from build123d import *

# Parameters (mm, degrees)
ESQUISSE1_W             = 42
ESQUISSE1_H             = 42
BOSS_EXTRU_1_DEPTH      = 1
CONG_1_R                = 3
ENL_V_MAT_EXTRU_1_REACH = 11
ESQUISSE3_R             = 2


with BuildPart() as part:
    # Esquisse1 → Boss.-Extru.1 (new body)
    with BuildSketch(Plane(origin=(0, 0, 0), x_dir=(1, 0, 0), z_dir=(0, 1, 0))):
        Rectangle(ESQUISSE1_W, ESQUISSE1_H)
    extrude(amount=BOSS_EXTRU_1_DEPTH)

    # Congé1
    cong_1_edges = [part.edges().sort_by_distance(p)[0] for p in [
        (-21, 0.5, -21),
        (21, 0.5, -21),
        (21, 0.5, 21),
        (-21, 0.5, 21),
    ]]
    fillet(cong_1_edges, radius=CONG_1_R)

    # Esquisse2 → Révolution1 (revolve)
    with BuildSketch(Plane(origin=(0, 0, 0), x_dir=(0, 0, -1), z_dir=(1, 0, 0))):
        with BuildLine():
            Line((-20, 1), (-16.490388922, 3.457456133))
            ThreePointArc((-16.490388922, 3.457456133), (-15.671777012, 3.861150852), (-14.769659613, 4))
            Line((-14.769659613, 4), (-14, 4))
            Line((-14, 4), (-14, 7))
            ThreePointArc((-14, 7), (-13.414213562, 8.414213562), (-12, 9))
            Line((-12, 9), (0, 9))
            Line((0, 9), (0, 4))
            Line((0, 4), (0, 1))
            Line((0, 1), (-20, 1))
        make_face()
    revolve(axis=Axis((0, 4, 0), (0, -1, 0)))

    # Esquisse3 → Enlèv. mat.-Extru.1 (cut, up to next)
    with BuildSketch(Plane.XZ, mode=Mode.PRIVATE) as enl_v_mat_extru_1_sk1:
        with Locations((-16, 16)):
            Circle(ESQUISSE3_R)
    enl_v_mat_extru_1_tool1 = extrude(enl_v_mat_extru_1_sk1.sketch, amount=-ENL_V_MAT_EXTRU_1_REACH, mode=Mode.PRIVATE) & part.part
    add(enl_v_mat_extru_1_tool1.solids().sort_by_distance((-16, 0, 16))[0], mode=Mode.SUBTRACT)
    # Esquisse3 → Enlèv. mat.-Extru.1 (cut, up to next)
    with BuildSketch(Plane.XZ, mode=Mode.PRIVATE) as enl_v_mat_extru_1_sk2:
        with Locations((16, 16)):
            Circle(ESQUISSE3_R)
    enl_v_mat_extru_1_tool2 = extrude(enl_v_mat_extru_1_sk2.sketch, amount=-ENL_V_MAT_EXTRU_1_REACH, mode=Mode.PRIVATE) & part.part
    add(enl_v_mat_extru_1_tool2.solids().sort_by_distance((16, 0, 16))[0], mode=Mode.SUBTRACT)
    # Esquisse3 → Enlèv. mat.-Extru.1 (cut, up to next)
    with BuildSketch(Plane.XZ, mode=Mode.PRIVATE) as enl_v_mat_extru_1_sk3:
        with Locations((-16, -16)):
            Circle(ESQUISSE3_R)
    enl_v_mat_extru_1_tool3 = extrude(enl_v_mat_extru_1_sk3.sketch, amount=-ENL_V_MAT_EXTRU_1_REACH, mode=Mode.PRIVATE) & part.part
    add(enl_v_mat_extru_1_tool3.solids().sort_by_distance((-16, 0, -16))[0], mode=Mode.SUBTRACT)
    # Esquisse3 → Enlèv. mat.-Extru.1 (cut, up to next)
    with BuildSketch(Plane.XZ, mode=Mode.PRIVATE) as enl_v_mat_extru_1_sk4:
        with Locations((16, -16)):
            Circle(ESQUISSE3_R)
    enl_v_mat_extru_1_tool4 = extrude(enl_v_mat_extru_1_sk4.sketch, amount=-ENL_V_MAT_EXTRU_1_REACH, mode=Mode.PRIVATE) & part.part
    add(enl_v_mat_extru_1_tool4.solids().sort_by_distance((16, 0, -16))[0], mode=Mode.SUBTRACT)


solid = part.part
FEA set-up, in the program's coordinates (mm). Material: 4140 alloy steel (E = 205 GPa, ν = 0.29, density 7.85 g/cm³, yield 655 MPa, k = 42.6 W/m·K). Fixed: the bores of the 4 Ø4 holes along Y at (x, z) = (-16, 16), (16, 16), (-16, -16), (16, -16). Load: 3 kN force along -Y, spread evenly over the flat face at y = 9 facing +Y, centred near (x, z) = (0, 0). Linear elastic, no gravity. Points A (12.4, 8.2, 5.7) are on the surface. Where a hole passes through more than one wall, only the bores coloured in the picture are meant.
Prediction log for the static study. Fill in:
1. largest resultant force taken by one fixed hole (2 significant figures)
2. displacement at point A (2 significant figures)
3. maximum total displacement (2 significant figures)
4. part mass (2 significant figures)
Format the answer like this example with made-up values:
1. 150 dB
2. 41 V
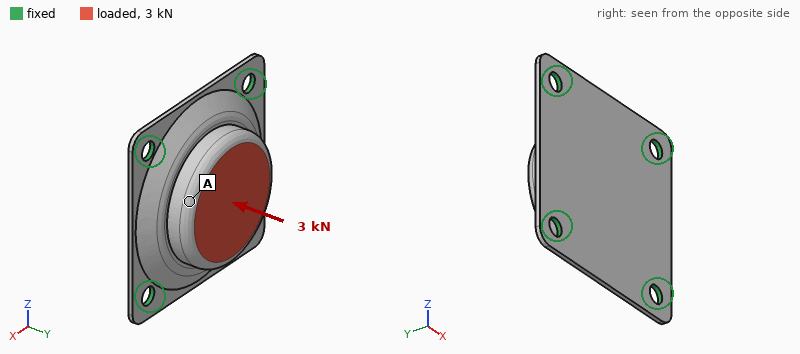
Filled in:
1. 1.3 kN
2. 17 µm
3. 18 µm
4. 61 g
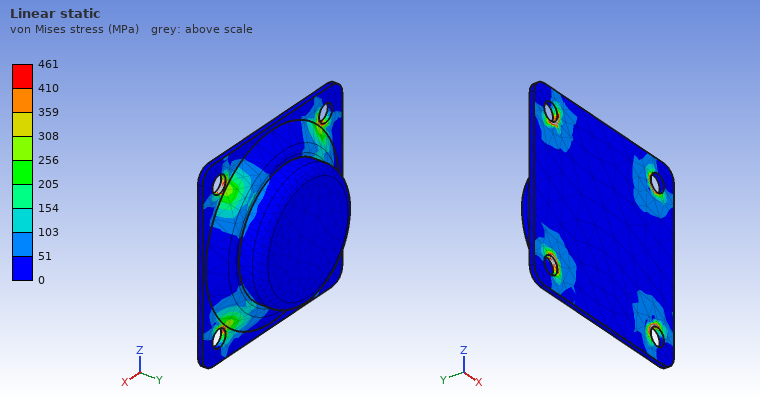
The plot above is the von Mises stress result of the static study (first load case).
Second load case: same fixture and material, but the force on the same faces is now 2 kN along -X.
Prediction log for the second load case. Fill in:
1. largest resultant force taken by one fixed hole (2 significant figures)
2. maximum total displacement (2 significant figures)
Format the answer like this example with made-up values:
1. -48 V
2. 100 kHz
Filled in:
1. 670 N
2. 8.9 µm
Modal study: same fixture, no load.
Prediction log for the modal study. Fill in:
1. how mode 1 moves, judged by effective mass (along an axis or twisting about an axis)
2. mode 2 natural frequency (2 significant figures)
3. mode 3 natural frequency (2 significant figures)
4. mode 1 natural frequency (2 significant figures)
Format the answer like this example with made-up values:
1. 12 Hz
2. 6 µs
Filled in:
1. along Y
2. 13 kHz
3. 13 kHz
4. 8900 Hz
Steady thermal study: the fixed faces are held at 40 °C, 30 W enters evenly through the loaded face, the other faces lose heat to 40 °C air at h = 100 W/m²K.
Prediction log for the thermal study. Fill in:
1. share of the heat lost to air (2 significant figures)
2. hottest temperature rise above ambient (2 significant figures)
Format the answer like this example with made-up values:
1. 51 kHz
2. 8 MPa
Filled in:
1. 39 %
2. 56 K
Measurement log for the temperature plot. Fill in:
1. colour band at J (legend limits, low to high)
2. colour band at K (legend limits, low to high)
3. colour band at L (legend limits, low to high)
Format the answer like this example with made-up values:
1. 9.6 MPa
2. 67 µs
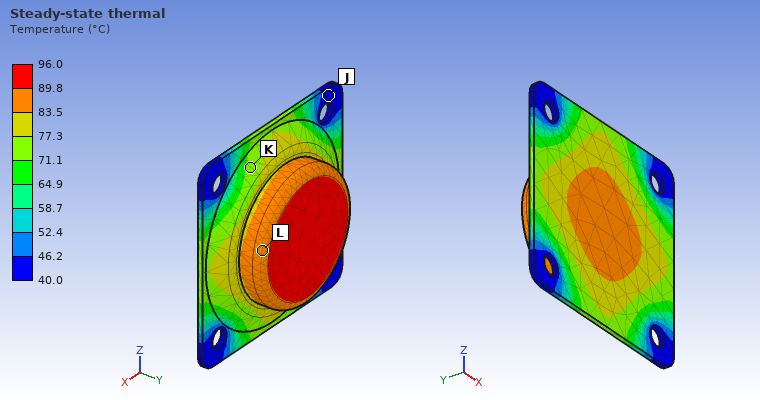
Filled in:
1. 40.0 to 46.2 °C
2. 71.1 to 77.3 °C
3. 83.5 to 89.8 °C
